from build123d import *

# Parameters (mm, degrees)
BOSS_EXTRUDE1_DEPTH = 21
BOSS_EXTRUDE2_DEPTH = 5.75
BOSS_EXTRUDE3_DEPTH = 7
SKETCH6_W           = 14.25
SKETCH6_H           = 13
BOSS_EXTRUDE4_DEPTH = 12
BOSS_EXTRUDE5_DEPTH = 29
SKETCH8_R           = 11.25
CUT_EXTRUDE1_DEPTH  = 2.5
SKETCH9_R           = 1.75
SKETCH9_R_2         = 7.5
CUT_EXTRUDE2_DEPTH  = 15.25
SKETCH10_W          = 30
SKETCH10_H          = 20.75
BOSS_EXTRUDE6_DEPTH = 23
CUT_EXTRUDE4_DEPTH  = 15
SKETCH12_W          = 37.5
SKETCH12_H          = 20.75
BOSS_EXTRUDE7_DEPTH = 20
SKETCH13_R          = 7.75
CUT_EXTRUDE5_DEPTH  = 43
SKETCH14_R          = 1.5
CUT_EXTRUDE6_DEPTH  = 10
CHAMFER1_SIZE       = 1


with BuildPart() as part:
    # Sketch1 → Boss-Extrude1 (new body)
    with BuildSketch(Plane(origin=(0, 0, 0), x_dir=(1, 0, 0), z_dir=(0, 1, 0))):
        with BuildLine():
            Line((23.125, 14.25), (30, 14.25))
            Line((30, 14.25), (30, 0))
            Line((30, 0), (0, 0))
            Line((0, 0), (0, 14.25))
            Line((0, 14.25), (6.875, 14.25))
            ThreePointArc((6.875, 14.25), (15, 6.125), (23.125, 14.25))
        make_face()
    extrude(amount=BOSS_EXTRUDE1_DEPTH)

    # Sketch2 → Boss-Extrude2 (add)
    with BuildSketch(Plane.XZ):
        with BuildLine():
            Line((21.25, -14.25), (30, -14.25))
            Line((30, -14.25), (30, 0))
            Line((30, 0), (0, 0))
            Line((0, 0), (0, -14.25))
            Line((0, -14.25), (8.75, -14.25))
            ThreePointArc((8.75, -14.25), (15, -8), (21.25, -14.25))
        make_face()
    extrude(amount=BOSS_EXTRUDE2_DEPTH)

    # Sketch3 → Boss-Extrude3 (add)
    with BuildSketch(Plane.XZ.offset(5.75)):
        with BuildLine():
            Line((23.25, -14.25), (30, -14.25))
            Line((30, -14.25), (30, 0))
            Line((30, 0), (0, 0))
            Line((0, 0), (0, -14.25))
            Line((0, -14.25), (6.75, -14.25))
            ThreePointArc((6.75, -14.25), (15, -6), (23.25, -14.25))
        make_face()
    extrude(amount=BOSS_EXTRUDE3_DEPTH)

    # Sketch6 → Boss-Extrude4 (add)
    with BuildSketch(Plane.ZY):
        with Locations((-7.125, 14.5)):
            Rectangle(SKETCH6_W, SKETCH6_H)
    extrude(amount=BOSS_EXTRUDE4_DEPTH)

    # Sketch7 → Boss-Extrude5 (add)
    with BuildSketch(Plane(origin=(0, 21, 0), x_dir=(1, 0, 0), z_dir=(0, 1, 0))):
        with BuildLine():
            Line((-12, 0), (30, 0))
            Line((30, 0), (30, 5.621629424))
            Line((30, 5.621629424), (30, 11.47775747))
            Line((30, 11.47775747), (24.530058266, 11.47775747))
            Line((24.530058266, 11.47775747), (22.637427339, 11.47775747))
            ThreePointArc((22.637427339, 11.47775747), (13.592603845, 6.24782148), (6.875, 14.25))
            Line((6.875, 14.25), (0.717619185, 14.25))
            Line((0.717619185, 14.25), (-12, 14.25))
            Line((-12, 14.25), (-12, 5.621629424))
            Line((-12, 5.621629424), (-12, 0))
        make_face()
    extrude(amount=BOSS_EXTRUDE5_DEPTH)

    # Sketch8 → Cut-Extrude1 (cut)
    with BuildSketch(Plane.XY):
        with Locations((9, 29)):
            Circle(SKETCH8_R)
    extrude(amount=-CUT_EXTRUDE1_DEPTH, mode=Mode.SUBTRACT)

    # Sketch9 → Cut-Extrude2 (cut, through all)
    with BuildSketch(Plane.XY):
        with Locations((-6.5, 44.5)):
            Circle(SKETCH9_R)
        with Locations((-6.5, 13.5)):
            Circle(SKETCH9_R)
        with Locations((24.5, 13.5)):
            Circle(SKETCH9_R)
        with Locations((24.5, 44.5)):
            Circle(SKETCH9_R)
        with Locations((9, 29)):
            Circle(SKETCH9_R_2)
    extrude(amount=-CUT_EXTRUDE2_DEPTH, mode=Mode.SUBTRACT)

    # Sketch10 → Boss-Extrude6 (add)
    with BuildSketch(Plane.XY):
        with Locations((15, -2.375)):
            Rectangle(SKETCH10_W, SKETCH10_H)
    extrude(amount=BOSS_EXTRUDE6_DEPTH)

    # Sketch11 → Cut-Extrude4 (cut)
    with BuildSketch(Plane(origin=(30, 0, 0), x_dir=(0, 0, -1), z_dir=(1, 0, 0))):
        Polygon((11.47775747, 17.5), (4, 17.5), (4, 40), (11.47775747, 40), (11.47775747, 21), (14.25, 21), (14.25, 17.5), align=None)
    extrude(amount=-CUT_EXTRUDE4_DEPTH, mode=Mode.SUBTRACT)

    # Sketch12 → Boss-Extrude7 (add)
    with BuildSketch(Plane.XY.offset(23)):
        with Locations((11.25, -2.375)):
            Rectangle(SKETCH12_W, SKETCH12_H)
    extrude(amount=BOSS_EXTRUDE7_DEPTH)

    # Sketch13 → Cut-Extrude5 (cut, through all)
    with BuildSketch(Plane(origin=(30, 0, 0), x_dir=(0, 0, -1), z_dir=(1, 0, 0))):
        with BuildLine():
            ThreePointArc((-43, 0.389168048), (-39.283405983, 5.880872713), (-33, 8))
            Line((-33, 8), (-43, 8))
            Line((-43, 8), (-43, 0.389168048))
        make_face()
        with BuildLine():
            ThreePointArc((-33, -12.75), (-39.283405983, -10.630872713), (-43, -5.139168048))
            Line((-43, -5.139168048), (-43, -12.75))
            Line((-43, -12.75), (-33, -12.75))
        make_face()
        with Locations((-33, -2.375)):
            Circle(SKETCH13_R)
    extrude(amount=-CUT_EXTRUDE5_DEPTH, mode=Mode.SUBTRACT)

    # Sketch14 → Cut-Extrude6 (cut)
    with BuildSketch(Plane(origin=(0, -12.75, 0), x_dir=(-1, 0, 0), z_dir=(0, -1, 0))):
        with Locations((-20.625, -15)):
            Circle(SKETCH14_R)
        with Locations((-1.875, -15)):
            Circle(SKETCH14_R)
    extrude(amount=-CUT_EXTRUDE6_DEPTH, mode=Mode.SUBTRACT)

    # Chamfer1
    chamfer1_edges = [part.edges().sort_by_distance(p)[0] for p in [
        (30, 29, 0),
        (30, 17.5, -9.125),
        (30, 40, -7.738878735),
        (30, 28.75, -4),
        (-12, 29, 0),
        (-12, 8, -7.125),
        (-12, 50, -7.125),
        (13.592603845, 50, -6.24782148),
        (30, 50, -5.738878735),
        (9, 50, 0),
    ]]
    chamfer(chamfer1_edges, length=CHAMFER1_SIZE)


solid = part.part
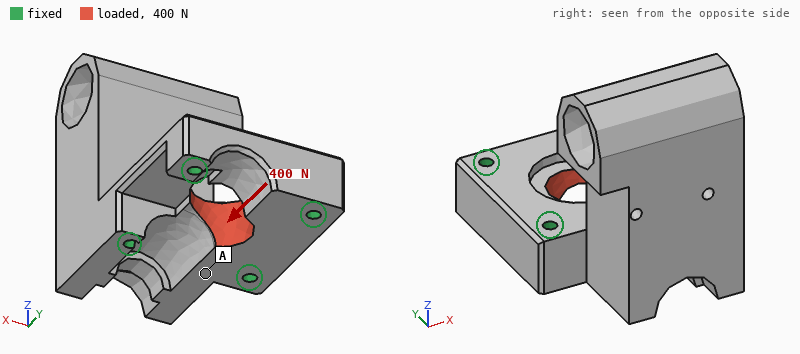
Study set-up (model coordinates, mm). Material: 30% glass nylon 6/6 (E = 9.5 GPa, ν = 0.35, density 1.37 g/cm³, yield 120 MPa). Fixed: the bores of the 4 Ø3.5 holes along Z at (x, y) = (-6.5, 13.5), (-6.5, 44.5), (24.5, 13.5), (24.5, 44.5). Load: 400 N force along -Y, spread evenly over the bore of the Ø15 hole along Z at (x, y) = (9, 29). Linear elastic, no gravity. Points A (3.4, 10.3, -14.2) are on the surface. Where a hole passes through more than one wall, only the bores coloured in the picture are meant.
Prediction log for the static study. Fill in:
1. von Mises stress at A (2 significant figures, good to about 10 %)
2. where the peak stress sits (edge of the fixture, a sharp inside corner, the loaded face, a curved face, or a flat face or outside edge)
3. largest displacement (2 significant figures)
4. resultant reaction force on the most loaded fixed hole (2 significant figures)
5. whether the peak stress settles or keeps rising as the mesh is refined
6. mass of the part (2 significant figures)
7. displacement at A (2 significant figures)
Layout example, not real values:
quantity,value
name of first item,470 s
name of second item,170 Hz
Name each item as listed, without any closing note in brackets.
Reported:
quantity,value
von Mises stress at A,0.27 MPa
where the peak stress sits,edge of the fixture
largest displacement,3.4 µm
resultant reaction force on the most loaded fixed hole,170 N
whether the peak stress settles or keeps rising as the mesh is refined,keeps rising
mass of the part,60 g
displacement at A,1.7 µm
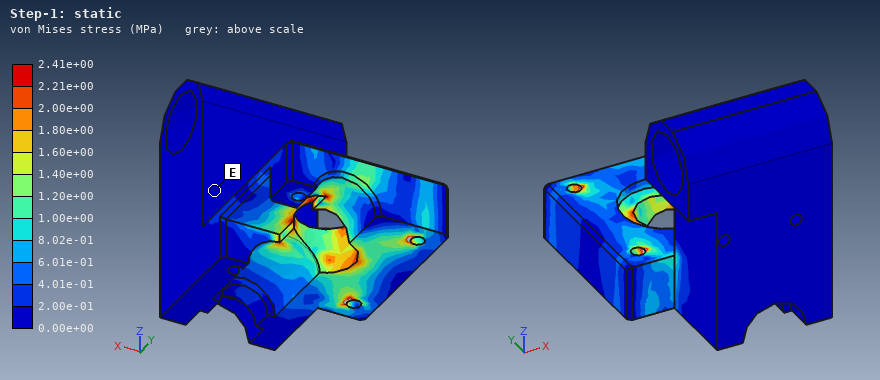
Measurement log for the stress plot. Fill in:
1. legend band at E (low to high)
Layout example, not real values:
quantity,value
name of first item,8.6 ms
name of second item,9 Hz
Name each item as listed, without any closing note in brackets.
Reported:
quantity,value
legend band at E,0.00e+00 to 2.00e-01 MPa
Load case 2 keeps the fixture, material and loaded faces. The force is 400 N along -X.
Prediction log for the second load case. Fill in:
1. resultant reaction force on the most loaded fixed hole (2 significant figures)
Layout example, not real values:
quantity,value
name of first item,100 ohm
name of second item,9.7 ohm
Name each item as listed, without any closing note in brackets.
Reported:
quantity,value
resultant reaction force on the most loaded fixed hole,170 N
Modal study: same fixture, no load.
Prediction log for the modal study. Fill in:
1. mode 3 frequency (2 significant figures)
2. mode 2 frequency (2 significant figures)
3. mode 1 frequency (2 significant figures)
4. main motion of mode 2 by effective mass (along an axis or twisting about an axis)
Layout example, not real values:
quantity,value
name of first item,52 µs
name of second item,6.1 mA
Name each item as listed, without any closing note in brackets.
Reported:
quantity,value
mode 3 frequency,5300 Hz
mode 2 frequency,2600 Hz
mode 1 frequency,1600 Hz
main motion of mode 2 by effective mass,along X
